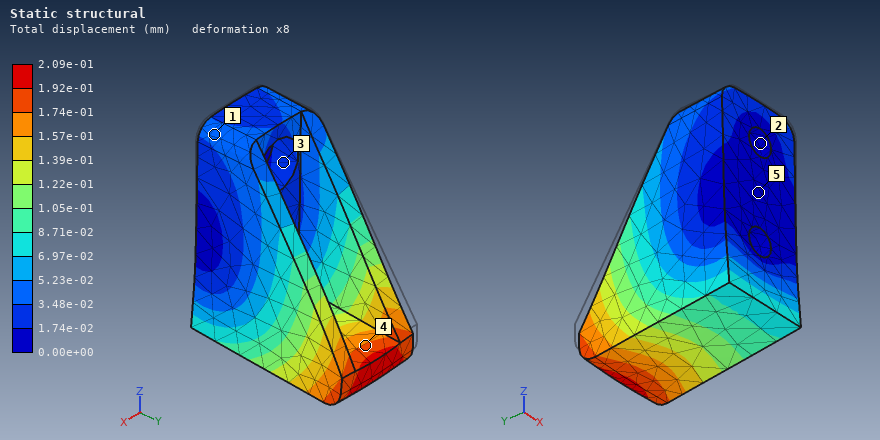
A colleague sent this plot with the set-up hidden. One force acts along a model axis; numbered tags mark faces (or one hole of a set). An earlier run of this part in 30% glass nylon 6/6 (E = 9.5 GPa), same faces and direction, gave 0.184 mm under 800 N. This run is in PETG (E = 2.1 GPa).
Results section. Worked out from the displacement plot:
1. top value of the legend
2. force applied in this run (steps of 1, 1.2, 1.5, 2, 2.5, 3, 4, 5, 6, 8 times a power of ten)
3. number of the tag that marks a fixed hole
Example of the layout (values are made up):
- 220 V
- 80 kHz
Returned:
- 2.09e-01 mm
- 200 N
- 2
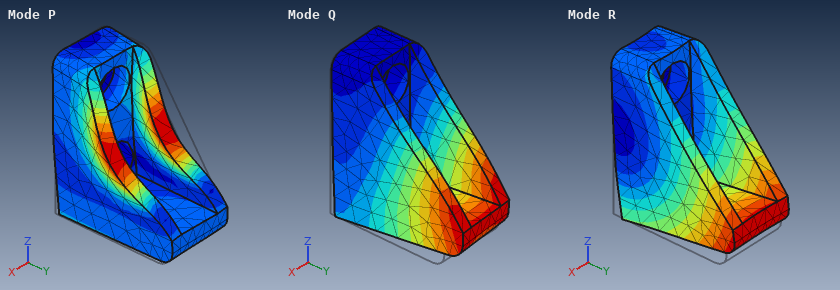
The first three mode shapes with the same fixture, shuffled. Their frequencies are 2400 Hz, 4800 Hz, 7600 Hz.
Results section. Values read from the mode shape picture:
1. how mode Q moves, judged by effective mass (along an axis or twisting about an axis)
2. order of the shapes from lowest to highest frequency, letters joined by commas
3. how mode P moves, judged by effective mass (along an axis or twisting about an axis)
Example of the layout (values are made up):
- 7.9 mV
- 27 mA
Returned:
- along X
- Q, R, P
- twisting about Y
